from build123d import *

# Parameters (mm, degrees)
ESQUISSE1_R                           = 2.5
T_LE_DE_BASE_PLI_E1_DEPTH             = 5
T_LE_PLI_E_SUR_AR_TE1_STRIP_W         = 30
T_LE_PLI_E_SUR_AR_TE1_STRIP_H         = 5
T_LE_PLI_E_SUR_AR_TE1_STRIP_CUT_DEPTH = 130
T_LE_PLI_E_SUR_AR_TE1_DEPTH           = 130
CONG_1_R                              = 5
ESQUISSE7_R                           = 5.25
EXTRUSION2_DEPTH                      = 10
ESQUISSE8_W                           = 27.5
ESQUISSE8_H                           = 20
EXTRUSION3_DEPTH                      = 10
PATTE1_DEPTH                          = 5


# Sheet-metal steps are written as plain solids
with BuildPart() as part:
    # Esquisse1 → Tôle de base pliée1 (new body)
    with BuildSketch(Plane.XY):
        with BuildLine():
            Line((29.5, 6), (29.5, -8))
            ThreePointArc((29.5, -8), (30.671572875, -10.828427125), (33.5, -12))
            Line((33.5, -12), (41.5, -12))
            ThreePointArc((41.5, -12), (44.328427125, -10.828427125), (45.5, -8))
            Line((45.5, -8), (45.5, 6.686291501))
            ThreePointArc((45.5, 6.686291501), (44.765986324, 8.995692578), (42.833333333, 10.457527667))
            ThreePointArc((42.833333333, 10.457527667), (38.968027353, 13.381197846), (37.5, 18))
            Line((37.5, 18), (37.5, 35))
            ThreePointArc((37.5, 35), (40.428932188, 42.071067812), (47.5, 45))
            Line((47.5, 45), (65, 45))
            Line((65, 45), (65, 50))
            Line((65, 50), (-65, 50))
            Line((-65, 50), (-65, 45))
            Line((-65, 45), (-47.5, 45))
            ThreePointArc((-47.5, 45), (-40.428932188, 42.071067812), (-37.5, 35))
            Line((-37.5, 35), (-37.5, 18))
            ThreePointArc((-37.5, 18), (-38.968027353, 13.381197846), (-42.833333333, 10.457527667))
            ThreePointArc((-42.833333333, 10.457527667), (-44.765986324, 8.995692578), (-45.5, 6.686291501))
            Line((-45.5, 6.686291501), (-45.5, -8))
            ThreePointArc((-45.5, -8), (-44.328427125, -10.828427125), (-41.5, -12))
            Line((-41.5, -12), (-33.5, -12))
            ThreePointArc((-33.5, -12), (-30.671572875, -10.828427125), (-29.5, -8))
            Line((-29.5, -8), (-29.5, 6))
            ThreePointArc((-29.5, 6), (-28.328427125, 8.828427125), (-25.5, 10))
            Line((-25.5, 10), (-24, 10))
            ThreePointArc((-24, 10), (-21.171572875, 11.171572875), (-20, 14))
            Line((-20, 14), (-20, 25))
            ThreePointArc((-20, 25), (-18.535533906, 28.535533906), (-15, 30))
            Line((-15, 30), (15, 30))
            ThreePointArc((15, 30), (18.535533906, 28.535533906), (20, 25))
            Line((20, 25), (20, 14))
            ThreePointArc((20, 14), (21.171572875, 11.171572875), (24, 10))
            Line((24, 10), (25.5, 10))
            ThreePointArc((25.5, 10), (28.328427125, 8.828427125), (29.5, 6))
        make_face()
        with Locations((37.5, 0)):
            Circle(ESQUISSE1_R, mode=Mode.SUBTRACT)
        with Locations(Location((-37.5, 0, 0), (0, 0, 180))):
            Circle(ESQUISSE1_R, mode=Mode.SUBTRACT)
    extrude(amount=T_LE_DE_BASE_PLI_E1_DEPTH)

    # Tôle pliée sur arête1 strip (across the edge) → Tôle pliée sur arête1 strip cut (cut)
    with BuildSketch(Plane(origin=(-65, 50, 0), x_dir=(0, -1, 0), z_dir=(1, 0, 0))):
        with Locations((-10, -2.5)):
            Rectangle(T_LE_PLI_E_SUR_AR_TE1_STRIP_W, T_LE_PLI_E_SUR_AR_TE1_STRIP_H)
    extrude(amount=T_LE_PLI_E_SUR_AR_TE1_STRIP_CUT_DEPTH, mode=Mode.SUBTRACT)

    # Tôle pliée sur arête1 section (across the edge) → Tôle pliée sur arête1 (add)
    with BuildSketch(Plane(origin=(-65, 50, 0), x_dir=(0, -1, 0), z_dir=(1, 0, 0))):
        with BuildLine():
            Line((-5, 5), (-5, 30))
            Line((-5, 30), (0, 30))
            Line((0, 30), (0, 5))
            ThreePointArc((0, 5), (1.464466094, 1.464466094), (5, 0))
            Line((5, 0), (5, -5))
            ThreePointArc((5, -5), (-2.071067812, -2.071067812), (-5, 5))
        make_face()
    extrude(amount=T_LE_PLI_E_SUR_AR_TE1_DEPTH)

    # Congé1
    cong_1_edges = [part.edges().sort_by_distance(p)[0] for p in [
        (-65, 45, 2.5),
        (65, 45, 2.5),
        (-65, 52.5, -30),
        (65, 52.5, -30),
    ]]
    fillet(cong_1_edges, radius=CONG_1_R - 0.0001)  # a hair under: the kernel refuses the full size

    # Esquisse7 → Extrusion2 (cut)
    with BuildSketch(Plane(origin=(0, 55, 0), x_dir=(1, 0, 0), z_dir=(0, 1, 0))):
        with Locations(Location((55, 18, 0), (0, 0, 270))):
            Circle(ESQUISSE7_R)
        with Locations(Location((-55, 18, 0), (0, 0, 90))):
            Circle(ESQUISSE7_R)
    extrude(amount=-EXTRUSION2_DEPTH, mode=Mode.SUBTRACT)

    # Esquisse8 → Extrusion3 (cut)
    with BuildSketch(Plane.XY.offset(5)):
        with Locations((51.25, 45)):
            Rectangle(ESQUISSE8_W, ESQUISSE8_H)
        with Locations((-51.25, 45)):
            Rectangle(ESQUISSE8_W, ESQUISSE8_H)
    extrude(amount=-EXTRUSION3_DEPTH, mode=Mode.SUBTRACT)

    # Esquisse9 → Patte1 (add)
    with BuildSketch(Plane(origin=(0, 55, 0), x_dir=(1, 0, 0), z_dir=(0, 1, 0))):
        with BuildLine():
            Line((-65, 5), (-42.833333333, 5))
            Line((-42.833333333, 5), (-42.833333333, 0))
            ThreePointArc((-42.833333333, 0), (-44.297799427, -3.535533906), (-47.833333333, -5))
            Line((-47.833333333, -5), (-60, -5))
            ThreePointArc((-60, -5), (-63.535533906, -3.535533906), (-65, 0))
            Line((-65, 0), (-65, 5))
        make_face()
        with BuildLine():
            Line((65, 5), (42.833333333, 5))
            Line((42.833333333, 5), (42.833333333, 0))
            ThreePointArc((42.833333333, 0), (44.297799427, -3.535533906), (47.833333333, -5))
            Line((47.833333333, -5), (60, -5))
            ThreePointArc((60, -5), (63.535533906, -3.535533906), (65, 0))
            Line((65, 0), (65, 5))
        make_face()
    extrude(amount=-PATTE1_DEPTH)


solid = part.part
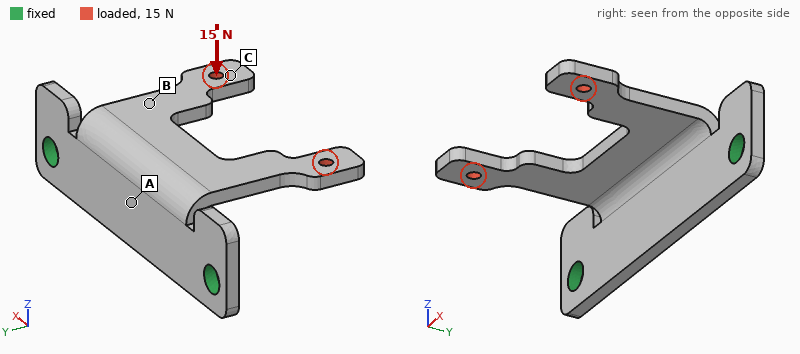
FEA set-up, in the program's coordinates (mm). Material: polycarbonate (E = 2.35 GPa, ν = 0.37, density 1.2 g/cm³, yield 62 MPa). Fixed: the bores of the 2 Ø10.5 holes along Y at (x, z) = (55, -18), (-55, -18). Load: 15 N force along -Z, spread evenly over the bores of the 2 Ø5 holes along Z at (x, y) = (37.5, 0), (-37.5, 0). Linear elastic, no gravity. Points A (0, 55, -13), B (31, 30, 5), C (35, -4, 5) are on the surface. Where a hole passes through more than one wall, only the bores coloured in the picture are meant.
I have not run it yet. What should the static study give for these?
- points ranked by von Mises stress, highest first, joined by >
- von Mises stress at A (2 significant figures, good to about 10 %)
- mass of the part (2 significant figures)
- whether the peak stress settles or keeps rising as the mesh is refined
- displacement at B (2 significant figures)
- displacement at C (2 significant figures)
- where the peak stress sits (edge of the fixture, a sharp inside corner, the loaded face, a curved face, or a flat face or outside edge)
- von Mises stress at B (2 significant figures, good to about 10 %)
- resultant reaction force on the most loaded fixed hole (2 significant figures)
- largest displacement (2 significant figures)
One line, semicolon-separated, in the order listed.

B > A > C; 0.99 MPa; 41 g; keeps rising; 0.48 mm; 1.5 mm; a sharp inside corner; 2.8 MPa; 7.7 N; 1.8 mm
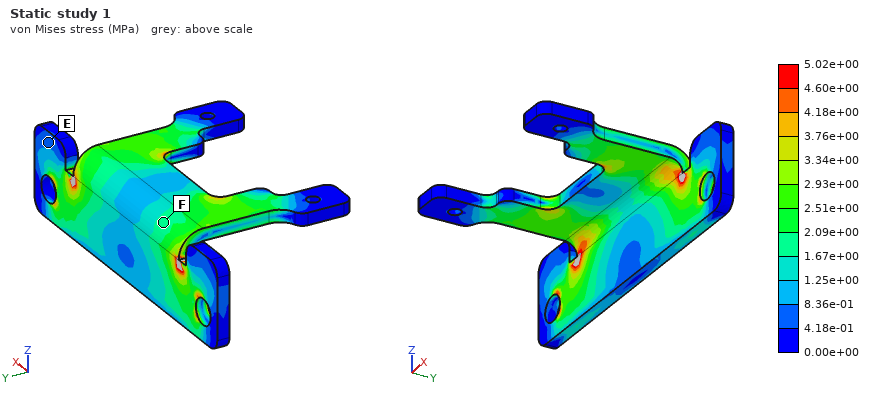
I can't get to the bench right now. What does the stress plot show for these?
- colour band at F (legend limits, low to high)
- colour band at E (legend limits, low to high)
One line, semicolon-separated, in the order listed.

1.67e+00 to 2.09e+00 MPa; 4.18e-01 to 8.36e-01 MPa
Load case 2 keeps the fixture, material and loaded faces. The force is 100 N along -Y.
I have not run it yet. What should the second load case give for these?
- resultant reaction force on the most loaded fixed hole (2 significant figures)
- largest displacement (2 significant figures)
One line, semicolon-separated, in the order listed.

50 N; 1.7 mm
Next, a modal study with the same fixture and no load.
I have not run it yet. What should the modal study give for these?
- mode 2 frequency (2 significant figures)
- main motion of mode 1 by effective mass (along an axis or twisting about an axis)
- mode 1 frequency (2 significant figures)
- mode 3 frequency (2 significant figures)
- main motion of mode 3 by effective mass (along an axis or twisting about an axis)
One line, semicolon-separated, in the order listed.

300 Hz; along Z; 210 Hz; 610 Hz; along Y
